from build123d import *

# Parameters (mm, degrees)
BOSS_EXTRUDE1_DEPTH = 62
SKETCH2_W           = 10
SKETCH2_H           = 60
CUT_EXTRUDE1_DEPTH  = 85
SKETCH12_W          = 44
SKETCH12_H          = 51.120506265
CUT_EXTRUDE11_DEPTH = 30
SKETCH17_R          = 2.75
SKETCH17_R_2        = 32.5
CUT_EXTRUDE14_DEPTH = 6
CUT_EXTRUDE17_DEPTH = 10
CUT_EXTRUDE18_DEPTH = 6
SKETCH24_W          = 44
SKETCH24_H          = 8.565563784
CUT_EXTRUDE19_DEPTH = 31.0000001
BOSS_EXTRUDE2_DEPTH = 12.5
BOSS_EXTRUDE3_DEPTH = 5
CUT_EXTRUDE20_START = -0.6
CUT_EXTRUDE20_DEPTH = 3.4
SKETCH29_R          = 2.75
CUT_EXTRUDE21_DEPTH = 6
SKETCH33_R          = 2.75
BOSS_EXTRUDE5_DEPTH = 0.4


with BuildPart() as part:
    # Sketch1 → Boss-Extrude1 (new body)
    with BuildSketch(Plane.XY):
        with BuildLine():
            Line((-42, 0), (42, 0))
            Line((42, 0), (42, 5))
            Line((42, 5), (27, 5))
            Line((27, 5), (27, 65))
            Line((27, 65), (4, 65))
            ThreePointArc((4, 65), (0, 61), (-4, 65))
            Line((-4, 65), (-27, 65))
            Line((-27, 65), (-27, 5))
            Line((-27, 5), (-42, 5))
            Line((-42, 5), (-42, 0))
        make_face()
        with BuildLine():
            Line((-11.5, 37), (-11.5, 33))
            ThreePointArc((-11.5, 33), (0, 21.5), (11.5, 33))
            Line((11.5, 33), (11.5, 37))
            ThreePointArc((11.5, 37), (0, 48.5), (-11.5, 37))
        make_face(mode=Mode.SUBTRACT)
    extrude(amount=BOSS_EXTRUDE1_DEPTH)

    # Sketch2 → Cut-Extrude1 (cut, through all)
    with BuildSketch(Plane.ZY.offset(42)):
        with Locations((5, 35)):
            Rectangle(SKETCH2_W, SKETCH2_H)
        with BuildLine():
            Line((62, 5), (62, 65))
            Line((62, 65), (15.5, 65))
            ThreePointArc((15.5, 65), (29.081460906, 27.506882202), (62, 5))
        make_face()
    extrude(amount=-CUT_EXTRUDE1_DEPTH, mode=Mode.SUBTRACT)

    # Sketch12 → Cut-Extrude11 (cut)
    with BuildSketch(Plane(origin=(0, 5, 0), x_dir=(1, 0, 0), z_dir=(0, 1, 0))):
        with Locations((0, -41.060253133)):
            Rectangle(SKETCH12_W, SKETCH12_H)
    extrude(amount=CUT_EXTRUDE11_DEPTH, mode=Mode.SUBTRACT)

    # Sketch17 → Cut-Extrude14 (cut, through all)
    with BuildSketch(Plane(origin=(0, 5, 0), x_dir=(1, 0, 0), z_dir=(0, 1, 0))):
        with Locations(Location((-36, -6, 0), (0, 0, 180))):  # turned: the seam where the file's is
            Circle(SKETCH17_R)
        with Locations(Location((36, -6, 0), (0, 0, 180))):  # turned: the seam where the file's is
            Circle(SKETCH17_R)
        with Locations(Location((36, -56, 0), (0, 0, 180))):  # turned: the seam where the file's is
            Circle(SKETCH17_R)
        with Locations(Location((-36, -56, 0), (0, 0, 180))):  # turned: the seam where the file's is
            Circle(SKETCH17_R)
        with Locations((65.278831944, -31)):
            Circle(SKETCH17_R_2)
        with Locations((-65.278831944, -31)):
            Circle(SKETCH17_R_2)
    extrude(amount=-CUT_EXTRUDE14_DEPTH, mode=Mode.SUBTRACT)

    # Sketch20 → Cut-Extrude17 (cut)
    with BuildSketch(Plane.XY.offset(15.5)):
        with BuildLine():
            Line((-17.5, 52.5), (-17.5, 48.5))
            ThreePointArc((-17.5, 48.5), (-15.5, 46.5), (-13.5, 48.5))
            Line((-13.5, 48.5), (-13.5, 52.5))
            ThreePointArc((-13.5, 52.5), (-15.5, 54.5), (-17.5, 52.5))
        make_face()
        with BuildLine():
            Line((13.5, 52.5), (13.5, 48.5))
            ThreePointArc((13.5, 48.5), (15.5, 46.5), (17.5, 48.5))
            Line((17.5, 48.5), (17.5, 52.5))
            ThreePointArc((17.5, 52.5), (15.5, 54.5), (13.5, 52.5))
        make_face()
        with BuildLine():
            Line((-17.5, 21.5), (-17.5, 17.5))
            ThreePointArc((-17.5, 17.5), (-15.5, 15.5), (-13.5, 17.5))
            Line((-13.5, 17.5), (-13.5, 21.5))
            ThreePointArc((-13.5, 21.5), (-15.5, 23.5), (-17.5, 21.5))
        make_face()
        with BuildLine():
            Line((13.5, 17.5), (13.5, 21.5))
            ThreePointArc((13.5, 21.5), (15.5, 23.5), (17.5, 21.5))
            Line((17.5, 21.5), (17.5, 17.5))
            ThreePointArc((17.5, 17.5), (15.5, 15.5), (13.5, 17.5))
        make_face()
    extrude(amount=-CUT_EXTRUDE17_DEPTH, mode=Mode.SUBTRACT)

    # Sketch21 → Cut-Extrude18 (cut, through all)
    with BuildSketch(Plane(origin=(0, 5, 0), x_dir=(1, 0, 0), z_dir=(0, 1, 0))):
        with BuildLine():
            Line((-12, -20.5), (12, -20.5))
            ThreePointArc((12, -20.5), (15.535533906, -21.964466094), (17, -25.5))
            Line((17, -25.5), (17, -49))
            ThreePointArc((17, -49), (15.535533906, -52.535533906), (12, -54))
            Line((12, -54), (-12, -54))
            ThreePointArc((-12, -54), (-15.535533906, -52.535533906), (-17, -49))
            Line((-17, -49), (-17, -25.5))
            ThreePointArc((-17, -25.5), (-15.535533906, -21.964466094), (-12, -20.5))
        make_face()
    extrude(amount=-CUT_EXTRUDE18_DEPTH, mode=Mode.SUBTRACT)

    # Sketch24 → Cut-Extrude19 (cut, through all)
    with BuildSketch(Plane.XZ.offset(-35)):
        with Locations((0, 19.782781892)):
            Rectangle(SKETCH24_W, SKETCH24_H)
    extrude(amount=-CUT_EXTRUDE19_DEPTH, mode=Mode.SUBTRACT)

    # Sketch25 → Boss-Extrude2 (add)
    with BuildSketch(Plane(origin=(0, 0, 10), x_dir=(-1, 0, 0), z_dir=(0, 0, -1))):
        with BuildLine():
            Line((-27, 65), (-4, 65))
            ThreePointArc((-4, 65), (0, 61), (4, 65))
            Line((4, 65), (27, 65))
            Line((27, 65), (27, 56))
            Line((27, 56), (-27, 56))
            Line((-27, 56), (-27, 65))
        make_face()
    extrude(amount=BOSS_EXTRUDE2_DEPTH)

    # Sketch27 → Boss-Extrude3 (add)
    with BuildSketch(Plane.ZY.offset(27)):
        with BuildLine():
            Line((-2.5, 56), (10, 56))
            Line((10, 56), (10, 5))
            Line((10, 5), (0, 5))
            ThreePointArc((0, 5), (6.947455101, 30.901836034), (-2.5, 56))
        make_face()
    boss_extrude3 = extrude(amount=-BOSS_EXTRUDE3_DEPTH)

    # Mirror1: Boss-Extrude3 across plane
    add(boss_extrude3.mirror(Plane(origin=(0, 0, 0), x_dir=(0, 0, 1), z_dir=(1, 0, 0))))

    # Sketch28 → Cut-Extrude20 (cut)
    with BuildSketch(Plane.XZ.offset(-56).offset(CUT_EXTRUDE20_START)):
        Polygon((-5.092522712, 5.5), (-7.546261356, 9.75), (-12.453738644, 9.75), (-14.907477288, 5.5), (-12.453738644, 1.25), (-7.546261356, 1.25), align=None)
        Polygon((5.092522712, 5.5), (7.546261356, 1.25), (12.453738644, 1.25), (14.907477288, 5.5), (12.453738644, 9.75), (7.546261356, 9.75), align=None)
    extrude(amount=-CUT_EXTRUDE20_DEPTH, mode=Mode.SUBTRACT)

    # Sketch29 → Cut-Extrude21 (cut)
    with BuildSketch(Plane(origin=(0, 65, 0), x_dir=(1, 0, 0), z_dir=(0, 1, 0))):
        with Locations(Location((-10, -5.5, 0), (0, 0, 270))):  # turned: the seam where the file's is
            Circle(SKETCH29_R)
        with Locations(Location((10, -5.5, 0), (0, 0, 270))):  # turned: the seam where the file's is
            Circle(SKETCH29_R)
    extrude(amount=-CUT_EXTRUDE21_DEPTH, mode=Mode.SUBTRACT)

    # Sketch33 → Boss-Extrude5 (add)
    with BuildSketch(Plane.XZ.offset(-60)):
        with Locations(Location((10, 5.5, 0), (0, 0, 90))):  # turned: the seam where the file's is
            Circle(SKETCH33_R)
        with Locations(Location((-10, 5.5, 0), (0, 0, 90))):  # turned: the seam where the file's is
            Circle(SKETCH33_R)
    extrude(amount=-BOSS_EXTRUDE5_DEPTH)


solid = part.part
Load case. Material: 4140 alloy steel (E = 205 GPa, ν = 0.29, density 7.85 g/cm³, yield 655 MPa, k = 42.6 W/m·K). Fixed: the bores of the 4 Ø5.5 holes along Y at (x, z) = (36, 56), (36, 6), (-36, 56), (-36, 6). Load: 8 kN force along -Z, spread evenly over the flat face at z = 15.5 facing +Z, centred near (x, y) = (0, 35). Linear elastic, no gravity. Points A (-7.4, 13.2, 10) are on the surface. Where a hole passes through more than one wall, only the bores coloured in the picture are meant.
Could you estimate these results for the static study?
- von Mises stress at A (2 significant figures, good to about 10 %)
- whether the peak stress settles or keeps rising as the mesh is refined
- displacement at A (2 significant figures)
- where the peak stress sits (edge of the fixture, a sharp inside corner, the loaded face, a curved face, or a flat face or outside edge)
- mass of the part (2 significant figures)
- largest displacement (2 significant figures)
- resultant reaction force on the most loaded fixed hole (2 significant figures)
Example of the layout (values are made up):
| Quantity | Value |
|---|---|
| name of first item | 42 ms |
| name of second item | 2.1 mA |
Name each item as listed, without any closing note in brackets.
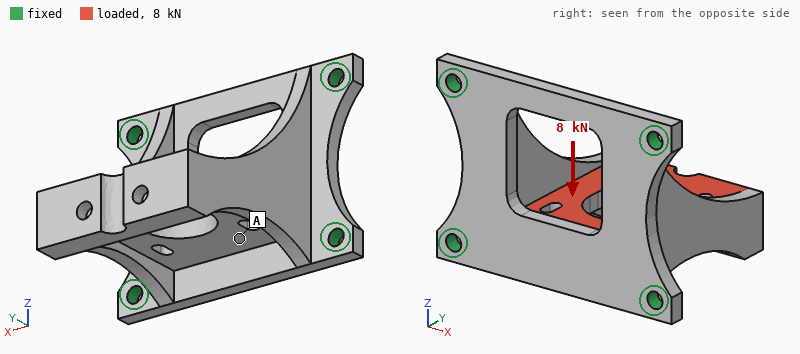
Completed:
| Quantity | Value |
|---|---|
| von Mises stress at A | 30 MPa |
| whether the peak stress settles or keeps rising as the mesh is refined | keeps rising |
| displacement at A | 0.030 mm |
| where the peak stress sits | edge of the fixture |
| mass of the part | 370 g |
| largest displacement | 0.17 mm |
| resultant reaction force on the most loaded fixed hole | 3.8 kN |
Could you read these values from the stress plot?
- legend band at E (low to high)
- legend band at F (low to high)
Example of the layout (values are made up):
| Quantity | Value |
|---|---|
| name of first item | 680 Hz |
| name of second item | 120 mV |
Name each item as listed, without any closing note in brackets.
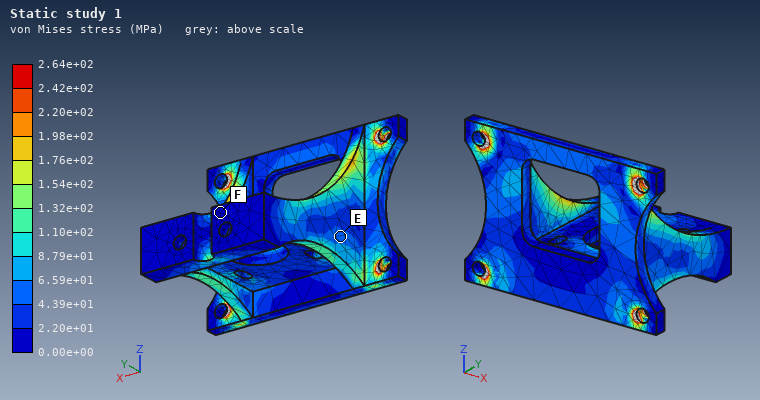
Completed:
| Quantity | Value |
|---|---|
| legend band at E | 4.39e+01 to 6.59e+01 MPa |
| legend band at F | 0.00e+00 to 2.20e+01 MPa |
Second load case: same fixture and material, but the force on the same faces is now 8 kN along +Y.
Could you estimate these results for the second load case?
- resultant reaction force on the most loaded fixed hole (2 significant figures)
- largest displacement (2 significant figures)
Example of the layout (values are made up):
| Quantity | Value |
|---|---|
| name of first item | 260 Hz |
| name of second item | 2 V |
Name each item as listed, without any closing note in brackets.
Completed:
| Quantity | Value |
|---|---|
| resultant reaction force on the most loaded fixed hole | 3.6 kN |
| largest displacement | 25 µm |
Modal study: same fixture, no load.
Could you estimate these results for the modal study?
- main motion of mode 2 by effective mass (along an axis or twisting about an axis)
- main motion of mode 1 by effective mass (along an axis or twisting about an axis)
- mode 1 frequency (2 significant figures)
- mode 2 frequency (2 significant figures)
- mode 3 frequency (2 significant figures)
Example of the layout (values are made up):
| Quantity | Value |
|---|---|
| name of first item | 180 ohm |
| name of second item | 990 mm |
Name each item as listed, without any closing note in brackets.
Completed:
| Quantity | Value |
|---|---|
| main motion of mode 2 by effective mass | along X |
| main motion of mode 1 by effective mass | along Z |
| mode 1 frequency | 2600 Hz |
| mode 2 frequency | 4000 Hz |
| mode 3 frequency | 4500 Hz |
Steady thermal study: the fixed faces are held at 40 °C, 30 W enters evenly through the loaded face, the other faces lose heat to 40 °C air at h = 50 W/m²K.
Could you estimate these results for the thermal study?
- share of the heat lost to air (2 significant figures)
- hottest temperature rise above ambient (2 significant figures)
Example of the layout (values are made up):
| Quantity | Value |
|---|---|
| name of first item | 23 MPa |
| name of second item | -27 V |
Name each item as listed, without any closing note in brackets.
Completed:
| Quantity | Value |
|---|---|
| share of the heat lost to air | 61 % |
| hottest temperature rise above ambient | 40 K |
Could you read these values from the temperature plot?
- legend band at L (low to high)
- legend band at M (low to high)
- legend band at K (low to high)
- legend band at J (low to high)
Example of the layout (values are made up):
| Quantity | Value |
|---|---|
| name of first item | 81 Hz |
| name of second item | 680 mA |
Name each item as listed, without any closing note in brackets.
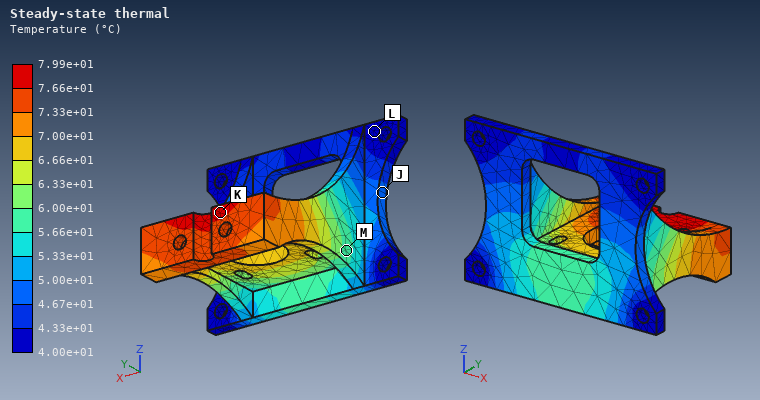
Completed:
| Quantity | Value |
|---|---|
| legend band at L | 4.00e+01 to 4.33e+01 °C |
| legend band at M | 5.66e+01 to 6.00e+01 °C |
| legend band at K | 7.66e+01 to 7.99e+01 °C |
| legend band at J | 4.67e+01 to 5.00e+01 °C |
